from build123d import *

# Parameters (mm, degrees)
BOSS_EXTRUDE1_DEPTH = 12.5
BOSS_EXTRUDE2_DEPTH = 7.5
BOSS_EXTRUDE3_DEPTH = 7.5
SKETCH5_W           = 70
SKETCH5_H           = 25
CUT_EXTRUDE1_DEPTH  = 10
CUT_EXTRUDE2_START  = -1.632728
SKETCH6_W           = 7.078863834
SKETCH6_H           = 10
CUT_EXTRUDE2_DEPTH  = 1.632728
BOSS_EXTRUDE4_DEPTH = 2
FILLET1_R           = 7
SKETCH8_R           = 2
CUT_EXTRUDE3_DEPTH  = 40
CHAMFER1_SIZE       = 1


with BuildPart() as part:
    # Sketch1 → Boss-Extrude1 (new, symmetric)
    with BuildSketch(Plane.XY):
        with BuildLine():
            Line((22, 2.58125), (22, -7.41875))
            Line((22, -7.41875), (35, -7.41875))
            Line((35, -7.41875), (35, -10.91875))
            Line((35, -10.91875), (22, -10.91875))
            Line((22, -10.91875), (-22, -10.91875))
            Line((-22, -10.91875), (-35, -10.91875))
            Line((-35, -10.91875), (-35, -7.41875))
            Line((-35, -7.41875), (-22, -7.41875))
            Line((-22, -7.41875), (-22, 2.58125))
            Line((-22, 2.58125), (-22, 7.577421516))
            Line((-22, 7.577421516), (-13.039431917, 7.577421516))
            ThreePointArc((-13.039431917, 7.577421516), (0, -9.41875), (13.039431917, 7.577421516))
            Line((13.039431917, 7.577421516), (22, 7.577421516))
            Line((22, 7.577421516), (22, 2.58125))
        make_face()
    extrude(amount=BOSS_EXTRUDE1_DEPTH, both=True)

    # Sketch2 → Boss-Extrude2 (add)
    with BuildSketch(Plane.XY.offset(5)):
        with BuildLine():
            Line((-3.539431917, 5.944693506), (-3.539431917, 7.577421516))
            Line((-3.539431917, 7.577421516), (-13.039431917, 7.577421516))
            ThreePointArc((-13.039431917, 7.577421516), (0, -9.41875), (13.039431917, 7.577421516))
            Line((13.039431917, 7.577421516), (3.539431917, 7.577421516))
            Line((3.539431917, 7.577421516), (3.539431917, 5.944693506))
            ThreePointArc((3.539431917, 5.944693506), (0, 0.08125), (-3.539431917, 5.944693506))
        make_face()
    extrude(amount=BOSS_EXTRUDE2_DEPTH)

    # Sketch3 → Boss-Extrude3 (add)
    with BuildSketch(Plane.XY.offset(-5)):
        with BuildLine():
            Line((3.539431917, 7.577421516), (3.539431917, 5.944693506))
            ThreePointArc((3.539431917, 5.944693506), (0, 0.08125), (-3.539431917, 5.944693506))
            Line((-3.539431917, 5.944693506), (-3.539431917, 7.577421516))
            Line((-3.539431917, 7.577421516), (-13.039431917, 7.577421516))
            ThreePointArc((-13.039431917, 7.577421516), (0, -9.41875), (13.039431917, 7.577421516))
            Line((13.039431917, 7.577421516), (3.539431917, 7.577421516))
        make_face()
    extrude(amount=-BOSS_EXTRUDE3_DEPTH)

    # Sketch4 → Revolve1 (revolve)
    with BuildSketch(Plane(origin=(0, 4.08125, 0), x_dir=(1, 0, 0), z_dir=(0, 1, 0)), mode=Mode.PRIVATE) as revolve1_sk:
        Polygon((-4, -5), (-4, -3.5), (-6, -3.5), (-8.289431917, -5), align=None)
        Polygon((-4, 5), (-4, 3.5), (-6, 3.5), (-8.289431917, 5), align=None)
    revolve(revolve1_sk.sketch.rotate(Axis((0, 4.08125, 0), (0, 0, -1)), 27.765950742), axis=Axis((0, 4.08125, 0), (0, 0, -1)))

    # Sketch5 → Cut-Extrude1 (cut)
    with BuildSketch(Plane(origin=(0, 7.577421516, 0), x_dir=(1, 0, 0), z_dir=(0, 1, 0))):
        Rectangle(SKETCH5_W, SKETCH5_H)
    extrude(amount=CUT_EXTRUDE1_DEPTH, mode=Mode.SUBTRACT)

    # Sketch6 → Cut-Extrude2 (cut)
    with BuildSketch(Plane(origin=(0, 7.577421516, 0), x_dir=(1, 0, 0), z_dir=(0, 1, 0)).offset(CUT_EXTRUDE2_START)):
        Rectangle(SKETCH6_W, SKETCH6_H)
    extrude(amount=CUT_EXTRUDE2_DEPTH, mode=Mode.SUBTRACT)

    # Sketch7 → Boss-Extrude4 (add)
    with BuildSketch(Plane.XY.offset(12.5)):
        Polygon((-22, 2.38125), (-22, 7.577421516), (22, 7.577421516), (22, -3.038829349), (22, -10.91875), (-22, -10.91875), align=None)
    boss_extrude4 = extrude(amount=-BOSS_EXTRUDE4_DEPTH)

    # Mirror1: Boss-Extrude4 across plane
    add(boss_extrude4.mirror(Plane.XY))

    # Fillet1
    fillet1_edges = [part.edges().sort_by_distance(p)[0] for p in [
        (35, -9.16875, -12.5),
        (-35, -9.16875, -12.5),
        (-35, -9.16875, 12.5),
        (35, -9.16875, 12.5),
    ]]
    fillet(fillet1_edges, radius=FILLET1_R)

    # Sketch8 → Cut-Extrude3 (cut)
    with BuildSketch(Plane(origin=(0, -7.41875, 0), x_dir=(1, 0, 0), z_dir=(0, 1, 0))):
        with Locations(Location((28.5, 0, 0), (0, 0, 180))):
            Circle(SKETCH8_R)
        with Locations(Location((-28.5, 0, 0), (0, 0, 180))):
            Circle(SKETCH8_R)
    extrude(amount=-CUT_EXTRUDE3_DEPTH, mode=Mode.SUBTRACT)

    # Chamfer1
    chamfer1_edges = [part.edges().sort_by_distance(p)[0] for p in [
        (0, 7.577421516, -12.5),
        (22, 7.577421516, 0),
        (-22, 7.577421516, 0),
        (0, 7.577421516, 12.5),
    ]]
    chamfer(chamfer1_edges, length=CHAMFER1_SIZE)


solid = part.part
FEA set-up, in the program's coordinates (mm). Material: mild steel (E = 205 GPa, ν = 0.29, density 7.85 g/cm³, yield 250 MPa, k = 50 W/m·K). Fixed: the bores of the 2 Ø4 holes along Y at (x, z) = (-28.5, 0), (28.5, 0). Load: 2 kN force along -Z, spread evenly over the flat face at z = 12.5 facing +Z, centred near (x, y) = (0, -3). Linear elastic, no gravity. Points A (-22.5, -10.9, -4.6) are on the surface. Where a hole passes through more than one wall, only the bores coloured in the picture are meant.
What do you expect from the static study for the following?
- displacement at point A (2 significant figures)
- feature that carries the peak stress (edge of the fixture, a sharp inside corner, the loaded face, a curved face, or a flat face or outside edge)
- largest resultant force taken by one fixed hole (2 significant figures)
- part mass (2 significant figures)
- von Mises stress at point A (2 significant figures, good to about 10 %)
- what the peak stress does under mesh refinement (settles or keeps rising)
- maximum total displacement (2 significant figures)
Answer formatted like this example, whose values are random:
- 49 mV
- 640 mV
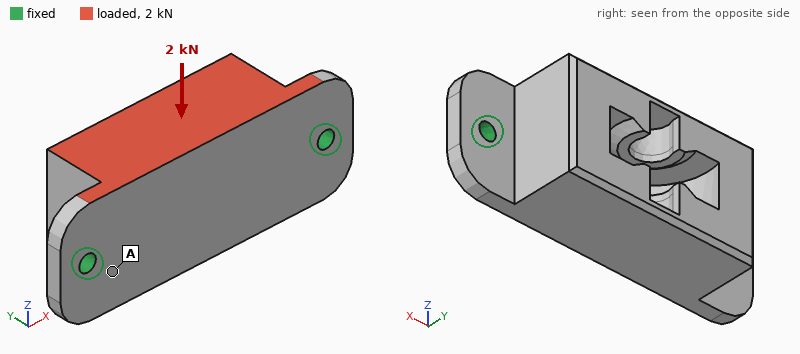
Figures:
- 6.2 µm
- edge of the fixture
- 1.0 kN
- 140 g
- 34 MPa
- keeps rising
- 37 µm
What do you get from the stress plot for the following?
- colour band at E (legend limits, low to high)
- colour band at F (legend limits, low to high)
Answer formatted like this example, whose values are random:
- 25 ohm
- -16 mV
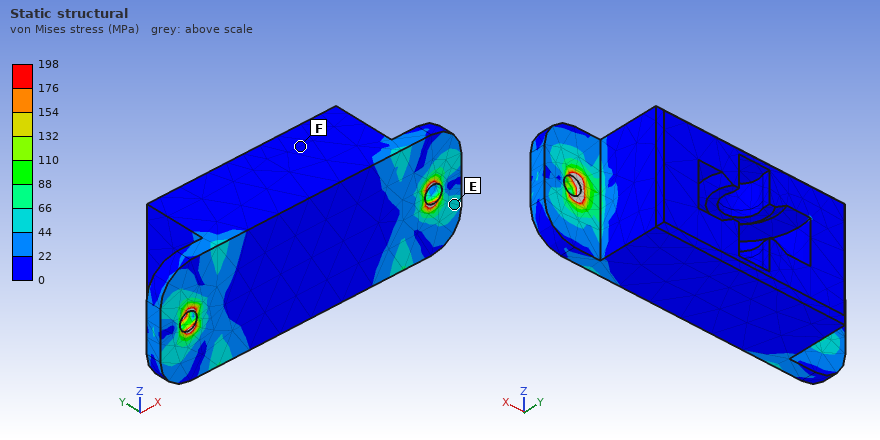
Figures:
- 44 to 66 MPa
- 0 to 22 MPa
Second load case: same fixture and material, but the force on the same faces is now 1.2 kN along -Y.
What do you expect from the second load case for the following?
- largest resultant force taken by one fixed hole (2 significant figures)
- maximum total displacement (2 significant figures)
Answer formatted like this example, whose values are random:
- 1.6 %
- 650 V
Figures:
- 720 N
- 40 µm
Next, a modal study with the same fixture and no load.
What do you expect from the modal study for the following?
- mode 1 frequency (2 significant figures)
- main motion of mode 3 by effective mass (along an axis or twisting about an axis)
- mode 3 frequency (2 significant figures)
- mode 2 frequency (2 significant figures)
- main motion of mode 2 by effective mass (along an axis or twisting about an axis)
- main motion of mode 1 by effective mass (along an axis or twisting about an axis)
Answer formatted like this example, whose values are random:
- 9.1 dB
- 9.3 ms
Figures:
- 3400 Hz
- along X
- 12 kHz
- 7600 Hz
- along Y
- along Z
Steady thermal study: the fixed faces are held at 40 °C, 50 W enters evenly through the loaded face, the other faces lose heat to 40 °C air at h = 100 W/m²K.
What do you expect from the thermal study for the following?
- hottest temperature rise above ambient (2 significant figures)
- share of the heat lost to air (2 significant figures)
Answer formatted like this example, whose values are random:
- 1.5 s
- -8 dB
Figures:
- 66 K
- 45 %
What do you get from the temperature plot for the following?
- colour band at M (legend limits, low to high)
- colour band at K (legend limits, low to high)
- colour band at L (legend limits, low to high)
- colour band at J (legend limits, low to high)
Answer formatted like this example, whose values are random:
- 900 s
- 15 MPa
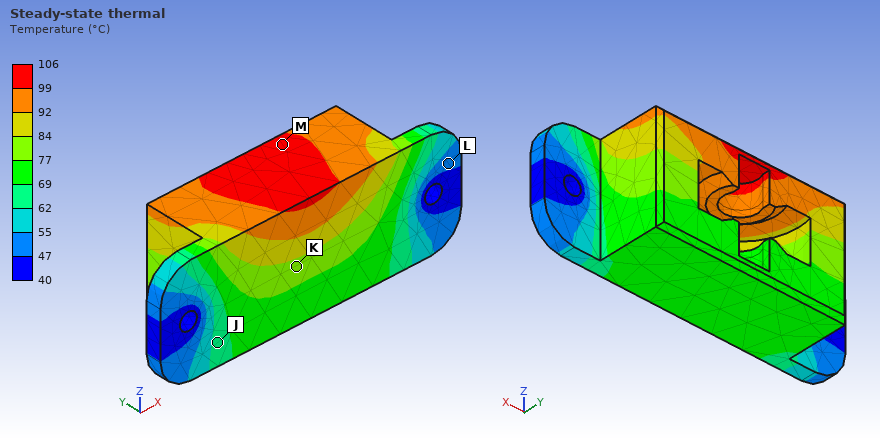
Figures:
- 99 to 106 °C
- 77 to 84 °C
- 47 to 55 °C
- 62 to 69 °C
